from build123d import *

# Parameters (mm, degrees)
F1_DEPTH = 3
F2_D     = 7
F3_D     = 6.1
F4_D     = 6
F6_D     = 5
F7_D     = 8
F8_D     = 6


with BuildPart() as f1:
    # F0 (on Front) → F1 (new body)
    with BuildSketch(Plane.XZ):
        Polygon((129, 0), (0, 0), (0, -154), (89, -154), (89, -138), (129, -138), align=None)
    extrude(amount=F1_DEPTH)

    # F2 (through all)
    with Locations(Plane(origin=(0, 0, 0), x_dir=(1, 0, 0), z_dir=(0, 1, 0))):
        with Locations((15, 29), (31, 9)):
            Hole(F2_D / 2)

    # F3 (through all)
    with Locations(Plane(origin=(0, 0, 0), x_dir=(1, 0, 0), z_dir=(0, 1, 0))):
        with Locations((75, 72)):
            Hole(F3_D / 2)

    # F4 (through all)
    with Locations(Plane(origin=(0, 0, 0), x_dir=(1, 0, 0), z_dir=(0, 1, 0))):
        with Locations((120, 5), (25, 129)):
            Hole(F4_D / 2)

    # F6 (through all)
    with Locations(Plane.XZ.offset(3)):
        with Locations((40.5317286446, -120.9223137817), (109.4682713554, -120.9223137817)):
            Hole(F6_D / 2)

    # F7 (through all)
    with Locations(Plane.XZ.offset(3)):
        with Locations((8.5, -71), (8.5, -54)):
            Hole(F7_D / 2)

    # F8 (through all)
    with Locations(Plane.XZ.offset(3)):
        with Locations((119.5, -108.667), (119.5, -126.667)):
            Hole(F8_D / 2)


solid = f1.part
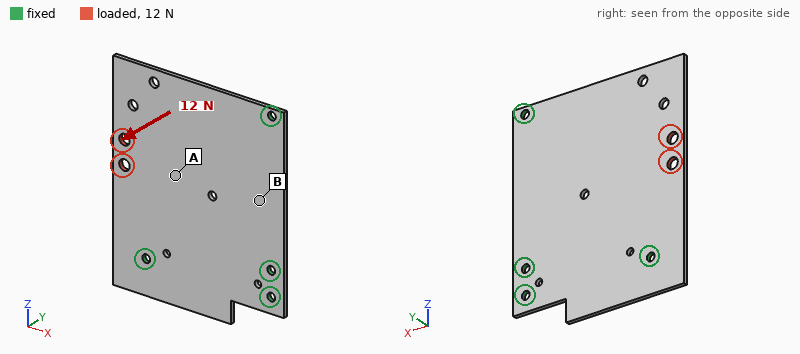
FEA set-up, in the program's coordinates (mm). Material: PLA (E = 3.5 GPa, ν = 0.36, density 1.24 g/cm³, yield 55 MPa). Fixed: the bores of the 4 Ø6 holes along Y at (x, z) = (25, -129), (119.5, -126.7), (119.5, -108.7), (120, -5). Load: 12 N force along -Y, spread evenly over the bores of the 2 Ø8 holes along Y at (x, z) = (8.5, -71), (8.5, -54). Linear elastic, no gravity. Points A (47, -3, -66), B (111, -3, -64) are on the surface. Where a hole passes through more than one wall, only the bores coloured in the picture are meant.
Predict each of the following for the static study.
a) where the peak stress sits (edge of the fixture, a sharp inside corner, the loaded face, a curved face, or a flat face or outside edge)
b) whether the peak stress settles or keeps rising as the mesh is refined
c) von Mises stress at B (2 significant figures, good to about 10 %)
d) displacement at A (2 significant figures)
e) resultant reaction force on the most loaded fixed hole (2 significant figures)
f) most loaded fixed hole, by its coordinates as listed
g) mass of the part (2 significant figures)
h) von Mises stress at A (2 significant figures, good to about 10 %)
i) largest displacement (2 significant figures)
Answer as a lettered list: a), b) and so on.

a) edge of the fixture
b) keeps rising
c) 0.76 MPa
d) 0.67 mm
e) 11 N
f) (25, -129)
g) 70 g
h) 2.0 MPa
i) 2.3 mm
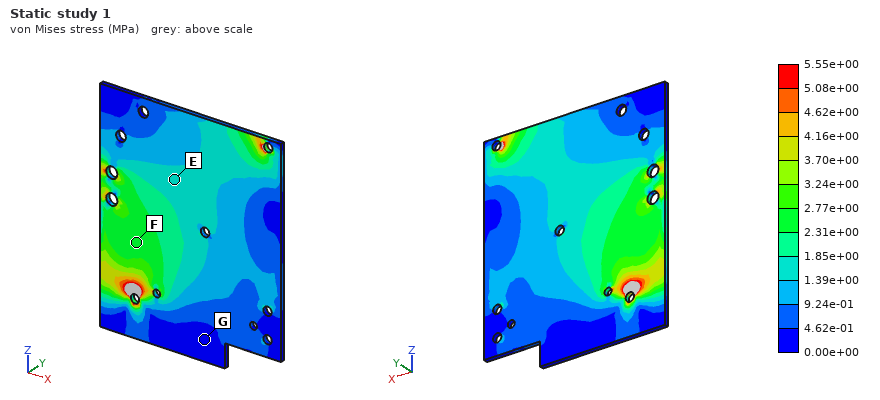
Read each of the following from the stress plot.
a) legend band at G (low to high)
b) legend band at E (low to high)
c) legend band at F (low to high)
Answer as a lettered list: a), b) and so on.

a) 0.00e+00 to 4.62e-01 MPa
b) 1.39e+00 to 1.85e+00 MPa
c) 2.31e+00 to 2.77e+00 MPa
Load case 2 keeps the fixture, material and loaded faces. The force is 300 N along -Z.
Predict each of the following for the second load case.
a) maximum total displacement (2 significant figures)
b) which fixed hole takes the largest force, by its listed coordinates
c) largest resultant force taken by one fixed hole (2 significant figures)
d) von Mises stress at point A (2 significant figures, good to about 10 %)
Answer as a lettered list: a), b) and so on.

a) 64 µm
b) (25, -129)
c) 240 N
d) 0.55 MPa
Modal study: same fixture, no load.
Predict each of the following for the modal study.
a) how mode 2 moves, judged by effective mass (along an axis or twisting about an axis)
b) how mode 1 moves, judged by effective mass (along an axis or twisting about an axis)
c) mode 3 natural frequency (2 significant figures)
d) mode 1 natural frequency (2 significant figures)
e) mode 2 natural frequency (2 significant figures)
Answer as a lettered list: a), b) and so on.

a) along Y
b) along Y
c) 360 Hz
d) 100 Hz
e) 330 Hz
